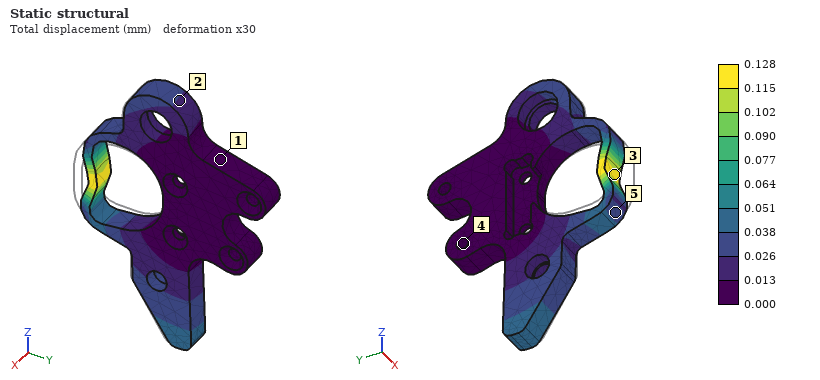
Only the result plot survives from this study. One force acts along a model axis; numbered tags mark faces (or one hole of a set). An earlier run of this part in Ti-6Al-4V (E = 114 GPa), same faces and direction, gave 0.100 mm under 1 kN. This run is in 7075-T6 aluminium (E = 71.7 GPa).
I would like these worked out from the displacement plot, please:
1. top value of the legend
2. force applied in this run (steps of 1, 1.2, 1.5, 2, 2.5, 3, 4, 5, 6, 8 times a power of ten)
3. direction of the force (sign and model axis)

0.128 mm
800 N
+Y
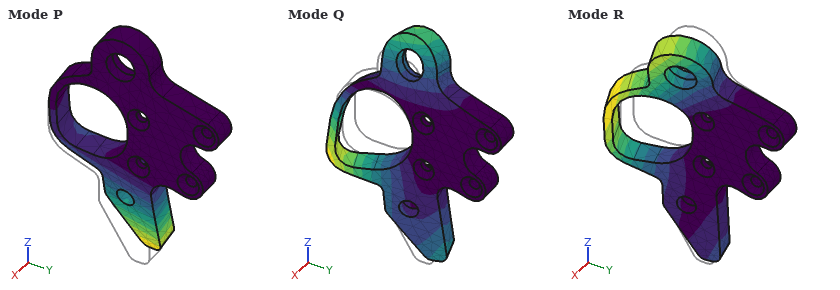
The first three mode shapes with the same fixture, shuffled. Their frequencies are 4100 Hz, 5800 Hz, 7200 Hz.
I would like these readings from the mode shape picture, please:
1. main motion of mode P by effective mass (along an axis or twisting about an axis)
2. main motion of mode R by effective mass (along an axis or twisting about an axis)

along X
along X
